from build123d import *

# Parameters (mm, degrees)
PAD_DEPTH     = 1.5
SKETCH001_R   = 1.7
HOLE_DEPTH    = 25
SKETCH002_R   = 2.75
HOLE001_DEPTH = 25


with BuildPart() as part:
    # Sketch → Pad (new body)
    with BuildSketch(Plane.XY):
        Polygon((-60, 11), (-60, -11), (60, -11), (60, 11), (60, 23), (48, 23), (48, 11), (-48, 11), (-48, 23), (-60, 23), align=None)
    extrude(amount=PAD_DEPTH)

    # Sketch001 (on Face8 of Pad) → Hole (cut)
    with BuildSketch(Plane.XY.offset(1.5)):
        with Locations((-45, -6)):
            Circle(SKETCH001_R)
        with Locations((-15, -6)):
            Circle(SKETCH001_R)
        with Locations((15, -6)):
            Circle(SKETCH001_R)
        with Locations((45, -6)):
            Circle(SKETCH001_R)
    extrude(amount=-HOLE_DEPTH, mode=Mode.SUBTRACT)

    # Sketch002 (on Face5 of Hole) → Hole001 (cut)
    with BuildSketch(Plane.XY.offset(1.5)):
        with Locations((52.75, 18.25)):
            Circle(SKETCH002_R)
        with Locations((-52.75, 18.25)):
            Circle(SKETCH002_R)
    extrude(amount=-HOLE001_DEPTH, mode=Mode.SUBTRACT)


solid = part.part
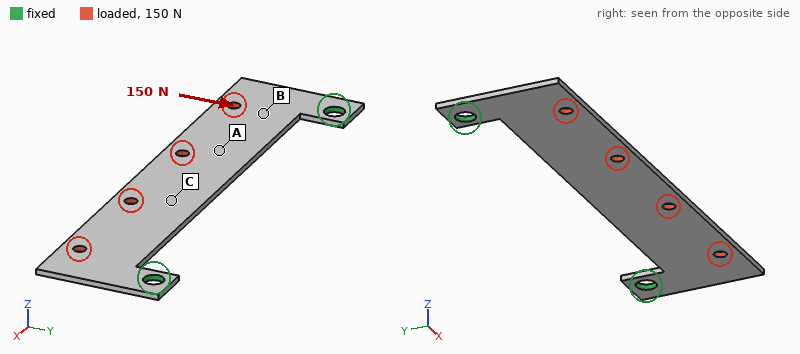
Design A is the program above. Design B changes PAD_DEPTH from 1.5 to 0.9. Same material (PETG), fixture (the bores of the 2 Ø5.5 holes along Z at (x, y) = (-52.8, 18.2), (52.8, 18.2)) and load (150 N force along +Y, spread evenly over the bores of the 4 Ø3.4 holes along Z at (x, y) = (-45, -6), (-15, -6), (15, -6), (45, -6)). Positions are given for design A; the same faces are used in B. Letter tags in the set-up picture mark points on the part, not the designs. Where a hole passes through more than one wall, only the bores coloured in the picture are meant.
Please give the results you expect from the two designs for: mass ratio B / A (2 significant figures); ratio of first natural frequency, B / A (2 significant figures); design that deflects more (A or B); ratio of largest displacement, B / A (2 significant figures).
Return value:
0.60
0.61
B
1.7
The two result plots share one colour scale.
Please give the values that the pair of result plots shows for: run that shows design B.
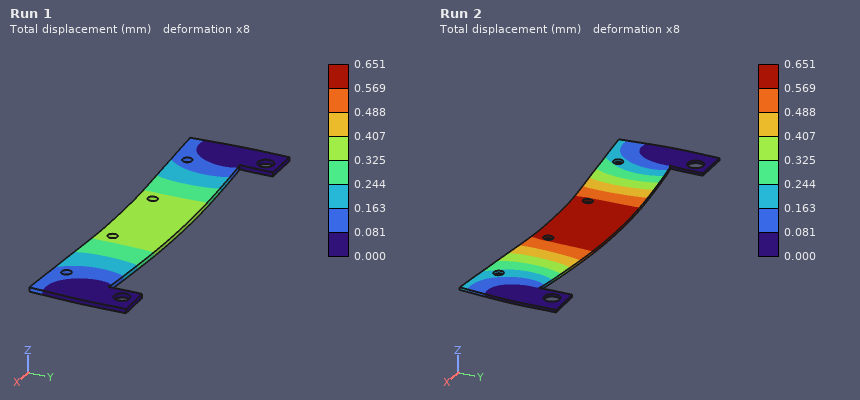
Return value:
Run 2
